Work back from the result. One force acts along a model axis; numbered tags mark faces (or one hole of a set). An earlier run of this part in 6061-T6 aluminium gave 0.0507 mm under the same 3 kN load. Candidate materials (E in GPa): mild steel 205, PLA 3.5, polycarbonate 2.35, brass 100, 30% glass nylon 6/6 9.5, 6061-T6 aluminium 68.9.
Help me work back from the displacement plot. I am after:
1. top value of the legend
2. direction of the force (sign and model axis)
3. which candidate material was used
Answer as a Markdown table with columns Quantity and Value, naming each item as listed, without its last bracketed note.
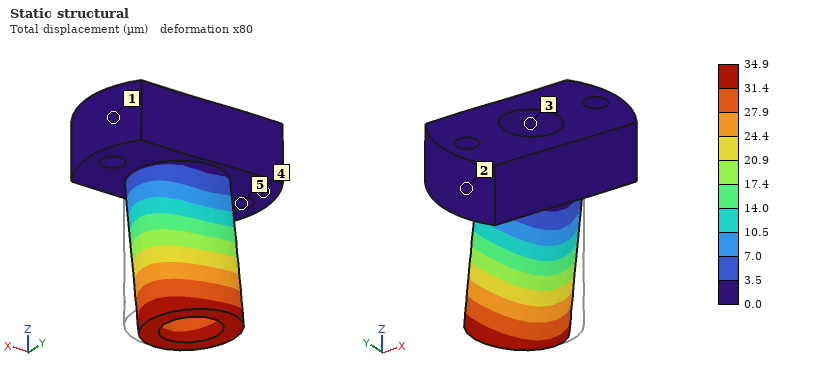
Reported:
| Quantity | Value |
|---|---|
| top value of the legend | 34.9 µm |
| direction of the force | -X |
| which candidate material was used | brass |
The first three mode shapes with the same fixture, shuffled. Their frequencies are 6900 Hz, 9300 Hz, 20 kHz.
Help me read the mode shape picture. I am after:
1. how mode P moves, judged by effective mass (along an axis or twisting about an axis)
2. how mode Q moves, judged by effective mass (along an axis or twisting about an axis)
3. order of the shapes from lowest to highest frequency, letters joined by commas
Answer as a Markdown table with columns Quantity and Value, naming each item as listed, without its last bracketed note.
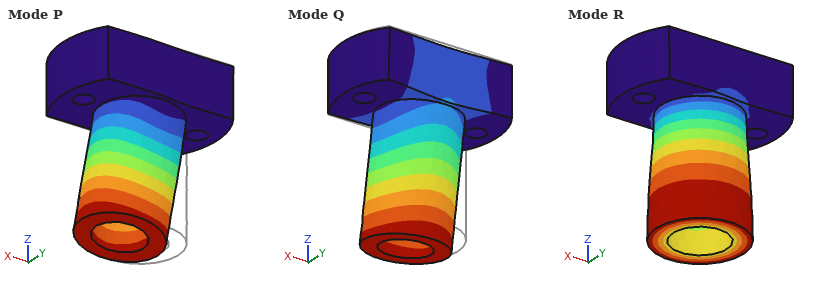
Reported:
| Quantity | Value |
|---|---|
| how mode P moves, judged by effective mass | along X |
| how mode Q moves, judged by effective mass | along Y |
| order of the shapes from lowest to highest frequency, letters joined by commas | Q, P, R |
